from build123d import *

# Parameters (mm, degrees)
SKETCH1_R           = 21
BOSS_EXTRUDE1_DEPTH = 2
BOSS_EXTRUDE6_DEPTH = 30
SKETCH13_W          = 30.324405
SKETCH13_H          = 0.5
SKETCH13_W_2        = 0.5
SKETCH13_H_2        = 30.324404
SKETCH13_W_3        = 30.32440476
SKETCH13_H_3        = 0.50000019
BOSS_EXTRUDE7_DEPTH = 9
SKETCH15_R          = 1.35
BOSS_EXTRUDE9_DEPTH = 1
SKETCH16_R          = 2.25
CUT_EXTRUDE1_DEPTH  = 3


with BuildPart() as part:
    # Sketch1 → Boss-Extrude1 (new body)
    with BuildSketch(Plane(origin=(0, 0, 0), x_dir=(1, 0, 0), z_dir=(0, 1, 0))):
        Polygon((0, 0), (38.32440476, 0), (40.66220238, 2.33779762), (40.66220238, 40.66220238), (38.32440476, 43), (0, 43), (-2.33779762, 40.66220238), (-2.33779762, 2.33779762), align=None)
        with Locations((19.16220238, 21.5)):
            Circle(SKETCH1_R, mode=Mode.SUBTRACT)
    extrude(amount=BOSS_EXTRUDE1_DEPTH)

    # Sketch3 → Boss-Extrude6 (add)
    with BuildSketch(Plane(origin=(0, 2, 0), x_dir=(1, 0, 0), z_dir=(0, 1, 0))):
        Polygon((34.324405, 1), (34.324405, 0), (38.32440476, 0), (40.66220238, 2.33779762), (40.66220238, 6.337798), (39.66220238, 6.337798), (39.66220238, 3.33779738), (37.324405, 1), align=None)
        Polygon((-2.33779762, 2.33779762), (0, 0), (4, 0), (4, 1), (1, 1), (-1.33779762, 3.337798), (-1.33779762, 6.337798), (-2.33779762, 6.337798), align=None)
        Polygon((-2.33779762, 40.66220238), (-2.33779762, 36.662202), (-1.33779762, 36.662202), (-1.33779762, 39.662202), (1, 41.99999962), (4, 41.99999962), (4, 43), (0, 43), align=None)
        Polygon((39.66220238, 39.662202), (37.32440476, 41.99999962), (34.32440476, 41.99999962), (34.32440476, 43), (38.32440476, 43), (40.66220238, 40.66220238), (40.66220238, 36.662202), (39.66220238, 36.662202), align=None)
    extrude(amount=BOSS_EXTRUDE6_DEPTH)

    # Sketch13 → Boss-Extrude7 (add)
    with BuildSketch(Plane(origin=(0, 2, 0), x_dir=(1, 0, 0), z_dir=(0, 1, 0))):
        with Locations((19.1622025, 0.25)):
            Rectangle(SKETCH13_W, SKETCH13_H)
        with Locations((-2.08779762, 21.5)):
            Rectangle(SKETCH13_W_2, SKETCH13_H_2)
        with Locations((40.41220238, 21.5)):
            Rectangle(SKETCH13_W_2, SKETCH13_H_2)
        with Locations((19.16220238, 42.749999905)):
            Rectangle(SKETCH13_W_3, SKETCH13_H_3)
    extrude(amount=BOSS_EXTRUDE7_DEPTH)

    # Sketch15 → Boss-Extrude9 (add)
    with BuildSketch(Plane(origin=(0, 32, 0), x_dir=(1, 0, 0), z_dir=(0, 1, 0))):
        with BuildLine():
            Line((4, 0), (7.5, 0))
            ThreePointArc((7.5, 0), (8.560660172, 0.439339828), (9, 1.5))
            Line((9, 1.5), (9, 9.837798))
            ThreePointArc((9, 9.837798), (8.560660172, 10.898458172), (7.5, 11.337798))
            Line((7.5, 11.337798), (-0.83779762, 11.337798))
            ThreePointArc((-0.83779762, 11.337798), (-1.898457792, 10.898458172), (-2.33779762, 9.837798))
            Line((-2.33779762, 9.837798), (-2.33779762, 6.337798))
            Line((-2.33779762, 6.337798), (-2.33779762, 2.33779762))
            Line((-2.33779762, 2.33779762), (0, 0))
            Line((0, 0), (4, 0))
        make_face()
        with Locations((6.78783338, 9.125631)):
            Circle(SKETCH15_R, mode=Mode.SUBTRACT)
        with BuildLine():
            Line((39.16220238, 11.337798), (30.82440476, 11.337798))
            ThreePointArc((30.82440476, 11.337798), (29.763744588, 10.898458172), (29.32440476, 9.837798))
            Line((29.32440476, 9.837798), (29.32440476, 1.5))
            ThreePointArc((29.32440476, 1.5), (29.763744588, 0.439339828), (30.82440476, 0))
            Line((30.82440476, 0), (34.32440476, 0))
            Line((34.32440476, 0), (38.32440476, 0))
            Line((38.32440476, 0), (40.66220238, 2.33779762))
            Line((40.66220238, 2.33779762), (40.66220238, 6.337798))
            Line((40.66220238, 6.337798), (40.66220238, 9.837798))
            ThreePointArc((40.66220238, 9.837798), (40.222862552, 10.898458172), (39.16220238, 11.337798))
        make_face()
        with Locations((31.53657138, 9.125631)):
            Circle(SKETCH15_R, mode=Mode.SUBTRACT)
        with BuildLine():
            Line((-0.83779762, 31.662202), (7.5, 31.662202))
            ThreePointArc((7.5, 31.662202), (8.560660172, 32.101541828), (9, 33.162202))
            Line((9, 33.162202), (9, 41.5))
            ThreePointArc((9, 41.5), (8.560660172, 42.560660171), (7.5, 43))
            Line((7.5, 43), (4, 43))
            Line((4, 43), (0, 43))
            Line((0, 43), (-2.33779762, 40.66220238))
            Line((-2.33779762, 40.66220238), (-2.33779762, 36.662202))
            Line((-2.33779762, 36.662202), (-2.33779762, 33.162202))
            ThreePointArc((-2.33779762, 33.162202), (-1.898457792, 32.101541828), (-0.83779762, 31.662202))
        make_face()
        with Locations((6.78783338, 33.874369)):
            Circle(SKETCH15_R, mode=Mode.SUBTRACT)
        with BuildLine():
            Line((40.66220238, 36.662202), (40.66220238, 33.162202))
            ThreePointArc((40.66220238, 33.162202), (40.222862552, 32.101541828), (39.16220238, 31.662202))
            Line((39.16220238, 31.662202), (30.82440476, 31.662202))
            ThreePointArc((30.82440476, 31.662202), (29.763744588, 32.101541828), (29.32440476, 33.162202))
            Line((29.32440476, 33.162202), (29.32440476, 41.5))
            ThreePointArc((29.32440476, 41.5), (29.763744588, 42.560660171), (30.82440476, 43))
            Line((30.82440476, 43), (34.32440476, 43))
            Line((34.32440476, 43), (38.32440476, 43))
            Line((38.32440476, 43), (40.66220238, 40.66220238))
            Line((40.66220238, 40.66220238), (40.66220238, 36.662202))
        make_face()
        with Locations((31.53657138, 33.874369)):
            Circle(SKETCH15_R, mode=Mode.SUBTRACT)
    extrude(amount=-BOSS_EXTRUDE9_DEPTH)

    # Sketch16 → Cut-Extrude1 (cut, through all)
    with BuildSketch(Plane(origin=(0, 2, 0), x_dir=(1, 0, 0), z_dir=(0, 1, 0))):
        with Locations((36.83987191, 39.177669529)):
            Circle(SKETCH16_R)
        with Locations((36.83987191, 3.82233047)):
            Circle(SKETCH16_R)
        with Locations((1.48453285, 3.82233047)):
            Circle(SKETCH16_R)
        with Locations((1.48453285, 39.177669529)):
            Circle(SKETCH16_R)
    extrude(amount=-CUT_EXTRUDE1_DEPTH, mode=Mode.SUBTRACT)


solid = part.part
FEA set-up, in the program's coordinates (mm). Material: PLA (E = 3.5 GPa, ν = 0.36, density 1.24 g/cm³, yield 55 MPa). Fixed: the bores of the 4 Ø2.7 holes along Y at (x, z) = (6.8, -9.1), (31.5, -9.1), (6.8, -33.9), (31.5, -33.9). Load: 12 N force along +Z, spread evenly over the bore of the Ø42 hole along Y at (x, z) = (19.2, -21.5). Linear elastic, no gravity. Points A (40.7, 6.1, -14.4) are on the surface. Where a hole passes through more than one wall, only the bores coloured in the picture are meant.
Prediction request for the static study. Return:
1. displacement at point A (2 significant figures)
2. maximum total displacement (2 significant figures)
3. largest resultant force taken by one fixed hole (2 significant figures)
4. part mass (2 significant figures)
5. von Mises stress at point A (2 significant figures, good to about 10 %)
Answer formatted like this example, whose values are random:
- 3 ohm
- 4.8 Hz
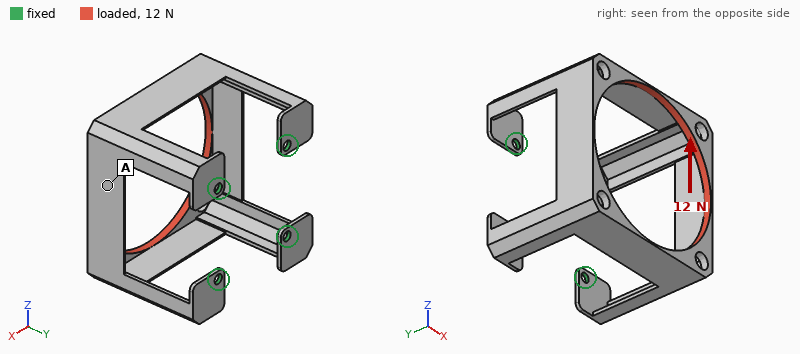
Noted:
- 0.54 mm
- 0.78 mm
- 6.2 N
- 3.9 g
- 3.1 MPa
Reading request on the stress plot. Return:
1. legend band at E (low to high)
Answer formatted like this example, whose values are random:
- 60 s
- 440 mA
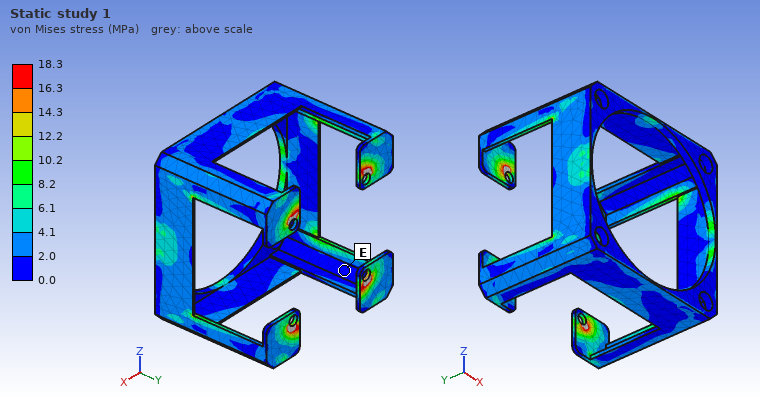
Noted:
- 0.0 to 2.0 MPa
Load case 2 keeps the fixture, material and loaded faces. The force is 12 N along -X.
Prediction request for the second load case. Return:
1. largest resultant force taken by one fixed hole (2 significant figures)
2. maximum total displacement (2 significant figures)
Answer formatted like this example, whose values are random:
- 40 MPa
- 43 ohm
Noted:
- 6.2 N
- 0.78 mm
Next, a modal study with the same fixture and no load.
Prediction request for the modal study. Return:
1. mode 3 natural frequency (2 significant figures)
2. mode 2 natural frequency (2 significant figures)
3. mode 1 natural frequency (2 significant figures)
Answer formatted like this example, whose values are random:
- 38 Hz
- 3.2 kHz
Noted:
- 450 Hz
- 440 Hz
- 440 Hz
